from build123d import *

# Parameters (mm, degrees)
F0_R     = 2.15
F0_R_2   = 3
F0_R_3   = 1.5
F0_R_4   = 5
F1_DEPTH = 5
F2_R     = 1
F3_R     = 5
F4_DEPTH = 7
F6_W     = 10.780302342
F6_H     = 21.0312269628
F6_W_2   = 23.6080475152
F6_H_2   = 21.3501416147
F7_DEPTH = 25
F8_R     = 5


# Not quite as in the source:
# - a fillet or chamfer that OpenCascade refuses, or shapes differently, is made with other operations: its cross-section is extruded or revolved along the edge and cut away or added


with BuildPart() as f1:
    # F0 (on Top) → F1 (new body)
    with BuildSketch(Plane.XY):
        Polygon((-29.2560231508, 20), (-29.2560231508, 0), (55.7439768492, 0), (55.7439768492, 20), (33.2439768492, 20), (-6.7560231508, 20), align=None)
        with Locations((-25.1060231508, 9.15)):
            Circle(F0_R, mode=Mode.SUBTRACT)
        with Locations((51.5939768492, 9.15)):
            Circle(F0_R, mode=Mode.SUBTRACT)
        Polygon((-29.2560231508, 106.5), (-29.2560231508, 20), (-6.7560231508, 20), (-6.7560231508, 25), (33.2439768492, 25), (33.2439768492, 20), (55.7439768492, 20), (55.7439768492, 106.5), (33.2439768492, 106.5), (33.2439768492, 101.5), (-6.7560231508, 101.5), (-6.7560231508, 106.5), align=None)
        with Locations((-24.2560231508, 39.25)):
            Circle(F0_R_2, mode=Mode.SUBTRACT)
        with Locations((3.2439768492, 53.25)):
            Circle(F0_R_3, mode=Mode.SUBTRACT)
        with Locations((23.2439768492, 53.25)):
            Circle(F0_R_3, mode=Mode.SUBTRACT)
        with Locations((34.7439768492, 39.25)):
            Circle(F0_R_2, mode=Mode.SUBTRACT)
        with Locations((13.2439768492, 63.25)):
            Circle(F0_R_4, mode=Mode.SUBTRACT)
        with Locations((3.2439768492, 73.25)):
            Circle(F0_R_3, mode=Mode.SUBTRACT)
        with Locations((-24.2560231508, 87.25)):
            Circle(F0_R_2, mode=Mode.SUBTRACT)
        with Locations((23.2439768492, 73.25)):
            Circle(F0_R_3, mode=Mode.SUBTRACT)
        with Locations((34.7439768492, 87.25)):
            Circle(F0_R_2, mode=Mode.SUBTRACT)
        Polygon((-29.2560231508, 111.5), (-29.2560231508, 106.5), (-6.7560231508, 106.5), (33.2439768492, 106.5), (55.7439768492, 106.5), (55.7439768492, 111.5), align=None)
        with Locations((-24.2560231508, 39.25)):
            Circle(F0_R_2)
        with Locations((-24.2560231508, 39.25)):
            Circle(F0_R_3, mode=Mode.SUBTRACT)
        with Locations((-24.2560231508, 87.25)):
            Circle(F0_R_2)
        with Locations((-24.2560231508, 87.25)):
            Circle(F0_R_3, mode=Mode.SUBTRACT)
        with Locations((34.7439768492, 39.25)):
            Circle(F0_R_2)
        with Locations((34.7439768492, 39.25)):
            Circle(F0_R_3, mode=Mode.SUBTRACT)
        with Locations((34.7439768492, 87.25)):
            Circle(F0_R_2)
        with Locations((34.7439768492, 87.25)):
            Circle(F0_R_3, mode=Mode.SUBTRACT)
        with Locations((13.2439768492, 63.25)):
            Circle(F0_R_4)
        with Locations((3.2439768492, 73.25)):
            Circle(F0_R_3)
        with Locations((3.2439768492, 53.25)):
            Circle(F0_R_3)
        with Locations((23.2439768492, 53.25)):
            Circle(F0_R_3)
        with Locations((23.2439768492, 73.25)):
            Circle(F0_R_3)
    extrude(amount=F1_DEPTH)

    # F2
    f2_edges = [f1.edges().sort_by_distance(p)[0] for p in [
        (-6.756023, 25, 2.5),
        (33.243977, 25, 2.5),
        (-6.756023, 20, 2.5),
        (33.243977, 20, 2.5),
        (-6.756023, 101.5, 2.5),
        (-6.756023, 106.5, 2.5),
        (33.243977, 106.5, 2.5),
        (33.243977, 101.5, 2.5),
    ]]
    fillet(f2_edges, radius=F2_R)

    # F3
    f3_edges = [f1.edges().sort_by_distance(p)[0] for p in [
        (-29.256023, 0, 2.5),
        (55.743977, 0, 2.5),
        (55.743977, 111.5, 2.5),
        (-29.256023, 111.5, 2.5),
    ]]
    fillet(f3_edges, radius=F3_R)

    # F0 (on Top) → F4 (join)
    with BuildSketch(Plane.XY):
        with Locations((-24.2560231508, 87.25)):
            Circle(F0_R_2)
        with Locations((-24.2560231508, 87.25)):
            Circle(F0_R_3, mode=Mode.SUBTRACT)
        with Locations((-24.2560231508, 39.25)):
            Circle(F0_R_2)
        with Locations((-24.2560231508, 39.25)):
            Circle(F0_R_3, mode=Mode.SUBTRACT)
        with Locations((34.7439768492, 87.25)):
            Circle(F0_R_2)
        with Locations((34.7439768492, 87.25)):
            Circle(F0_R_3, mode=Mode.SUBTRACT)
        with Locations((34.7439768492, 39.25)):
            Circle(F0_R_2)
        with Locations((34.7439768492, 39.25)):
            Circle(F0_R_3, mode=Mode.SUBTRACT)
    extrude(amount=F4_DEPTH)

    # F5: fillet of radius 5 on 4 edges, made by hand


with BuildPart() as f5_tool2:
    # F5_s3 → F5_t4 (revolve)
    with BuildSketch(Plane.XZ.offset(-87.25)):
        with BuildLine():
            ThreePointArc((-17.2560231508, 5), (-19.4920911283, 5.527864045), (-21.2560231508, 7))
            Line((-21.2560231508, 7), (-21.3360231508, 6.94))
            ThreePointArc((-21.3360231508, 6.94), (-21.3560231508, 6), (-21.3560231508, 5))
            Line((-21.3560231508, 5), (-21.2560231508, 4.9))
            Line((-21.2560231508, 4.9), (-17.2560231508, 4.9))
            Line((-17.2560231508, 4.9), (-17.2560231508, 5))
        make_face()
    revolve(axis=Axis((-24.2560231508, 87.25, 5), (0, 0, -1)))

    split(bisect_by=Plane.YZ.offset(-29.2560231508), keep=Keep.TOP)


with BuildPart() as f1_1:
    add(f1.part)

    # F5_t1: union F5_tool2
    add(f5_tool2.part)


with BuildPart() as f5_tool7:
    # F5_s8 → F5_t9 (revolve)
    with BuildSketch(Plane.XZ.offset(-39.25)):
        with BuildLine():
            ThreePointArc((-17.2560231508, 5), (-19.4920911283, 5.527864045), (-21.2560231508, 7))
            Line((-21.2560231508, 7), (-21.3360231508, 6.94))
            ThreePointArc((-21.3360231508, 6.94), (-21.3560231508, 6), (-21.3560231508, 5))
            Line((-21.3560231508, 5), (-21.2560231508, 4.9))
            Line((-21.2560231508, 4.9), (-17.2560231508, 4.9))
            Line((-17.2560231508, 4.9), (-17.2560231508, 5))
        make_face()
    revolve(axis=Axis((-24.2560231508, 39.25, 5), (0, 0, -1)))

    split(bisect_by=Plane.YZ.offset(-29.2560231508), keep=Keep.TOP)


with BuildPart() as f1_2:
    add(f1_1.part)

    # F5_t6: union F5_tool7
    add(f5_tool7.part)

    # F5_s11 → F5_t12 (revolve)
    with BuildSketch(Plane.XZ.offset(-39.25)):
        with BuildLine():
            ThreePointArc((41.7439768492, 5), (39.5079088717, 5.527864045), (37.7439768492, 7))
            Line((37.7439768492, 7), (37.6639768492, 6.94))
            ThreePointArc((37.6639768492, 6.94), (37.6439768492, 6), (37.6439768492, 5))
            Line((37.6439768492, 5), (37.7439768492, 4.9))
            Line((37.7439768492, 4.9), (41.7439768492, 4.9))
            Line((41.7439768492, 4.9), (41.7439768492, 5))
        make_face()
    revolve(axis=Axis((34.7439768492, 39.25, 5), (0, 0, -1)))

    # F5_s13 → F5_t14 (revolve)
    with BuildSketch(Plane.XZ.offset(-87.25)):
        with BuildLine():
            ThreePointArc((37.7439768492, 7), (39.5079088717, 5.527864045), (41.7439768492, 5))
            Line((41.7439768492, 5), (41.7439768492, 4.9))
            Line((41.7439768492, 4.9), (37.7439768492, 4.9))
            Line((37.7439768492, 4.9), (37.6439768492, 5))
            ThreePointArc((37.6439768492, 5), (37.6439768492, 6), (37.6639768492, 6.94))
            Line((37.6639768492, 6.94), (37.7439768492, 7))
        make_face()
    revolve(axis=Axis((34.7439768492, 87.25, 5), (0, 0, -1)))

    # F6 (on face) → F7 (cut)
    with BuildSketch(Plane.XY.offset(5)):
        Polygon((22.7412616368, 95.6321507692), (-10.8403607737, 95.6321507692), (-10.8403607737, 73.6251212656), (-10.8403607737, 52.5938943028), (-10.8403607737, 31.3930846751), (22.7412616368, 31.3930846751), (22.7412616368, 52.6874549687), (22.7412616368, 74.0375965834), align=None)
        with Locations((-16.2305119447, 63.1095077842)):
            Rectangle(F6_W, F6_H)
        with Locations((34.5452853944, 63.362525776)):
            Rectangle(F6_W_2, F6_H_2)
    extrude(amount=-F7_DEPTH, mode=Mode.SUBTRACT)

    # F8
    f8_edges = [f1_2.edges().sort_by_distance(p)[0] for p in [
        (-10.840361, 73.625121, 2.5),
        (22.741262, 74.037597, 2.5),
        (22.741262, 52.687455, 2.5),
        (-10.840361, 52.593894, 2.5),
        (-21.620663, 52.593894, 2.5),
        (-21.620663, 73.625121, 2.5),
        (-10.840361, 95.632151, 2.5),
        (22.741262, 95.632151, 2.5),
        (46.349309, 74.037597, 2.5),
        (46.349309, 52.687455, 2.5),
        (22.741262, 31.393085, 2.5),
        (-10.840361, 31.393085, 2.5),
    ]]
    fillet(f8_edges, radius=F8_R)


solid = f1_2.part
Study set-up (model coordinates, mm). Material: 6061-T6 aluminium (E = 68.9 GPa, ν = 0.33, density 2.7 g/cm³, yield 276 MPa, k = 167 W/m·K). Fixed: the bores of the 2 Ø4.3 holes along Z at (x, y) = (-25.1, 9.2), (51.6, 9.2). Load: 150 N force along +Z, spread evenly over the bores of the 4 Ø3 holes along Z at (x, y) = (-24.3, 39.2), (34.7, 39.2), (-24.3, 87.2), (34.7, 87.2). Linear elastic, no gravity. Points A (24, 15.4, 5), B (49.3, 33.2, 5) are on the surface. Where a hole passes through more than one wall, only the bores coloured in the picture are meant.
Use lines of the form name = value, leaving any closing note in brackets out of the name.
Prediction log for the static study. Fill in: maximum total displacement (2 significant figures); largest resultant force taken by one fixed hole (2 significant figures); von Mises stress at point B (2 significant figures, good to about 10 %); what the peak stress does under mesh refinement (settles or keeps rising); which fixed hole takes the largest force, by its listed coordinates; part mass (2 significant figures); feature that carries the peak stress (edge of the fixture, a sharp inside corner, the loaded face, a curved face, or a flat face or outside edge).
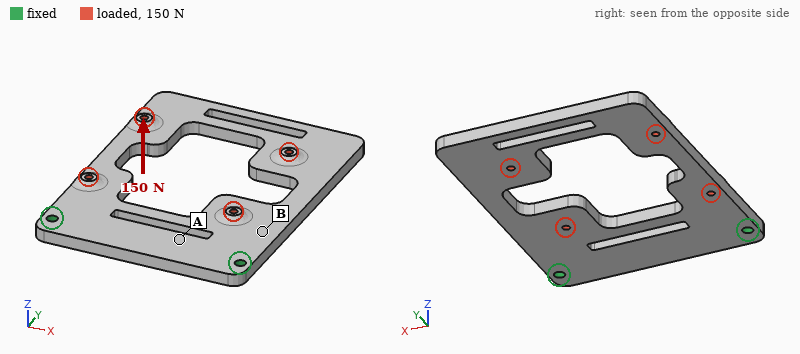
maximum total displacement = 0.86 mm
largest resultant force taken by one fixed hole = 89 N
von Mises stress at point B = 21 MPa
what the peak stress does under mesh refinement = keeps rising
which fixed hole takes the largest force, by its listed coordinates = (-25.1, 9.2)
part mass = 84 g
feature that carries the peak stress = edge of the fixture
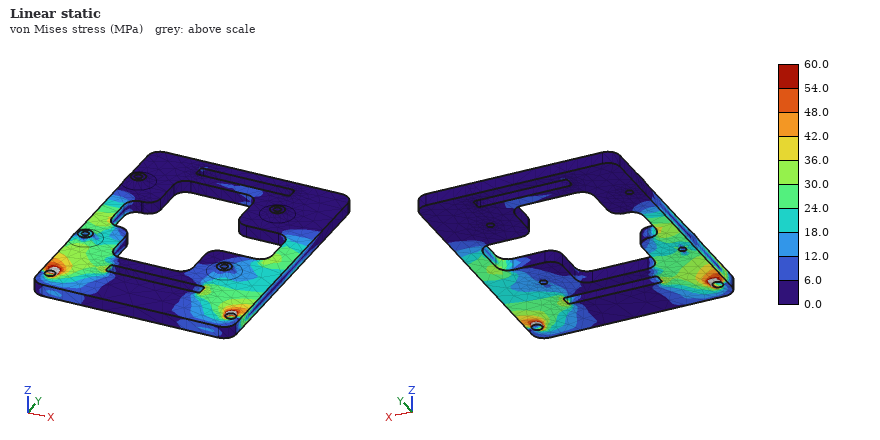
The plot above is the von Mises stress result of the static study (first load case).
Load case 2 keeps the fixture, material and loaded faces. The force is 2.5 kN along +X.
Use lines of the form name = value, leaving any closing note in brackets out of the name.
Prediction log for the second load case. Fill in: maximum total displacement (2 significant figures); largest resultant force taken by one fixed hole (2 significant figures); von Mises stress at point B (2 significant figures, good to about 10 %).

maximum total displacement = 0.37 mm
largest resultant force taken by one fixed hole = 2.1 kN
von Mises stress at point B = 28 MPa
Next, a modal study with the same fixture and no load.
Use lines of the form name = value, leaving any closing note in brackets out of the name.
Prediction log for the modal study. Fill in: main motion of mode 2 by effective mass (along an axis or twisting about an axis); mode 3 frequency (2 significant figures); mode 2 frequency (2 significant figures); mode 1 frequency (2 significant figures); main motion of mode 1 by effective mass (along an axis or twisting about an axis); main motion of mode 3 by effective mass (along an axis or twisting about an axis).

main motion of mode 2 by effective mass = twisting about Y
mode 3 frequency = 1800 Hz
mode 2 frequency = 800 Hz
mode 1 frequency = 300 Hz
main motion of mode 1 by effective mass = along Z
main motion of mode 3 by effective mass = along X
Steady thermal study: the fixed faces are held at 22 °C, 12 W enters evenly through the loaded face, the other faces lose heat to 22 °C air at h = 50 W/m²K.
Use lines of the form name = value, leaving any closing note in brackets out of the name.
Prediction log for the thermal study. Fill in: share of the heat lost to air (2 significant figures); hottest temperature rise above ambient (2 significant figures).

share of the heat lost to air = 45 %
hottest temperature rise above ambient = 13 K
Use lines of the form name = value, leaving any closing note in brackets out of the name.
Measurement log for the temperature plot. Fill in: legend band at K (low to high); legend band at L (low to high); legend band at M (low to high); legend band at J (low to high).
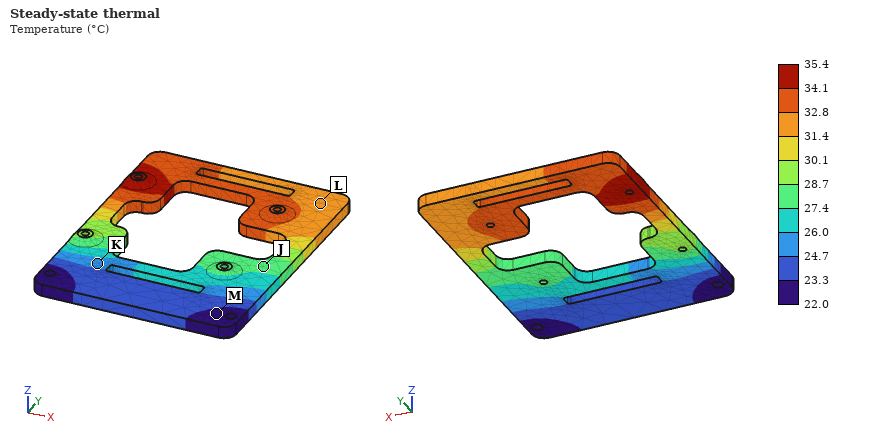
legend band at K = 24.7 to 26.0 °C
legend band at L = 31.4 to 32.8 °C
legend band at M = 22.0 to 23.3 °C
legend band at J = 27.4 to 28.7 °C
